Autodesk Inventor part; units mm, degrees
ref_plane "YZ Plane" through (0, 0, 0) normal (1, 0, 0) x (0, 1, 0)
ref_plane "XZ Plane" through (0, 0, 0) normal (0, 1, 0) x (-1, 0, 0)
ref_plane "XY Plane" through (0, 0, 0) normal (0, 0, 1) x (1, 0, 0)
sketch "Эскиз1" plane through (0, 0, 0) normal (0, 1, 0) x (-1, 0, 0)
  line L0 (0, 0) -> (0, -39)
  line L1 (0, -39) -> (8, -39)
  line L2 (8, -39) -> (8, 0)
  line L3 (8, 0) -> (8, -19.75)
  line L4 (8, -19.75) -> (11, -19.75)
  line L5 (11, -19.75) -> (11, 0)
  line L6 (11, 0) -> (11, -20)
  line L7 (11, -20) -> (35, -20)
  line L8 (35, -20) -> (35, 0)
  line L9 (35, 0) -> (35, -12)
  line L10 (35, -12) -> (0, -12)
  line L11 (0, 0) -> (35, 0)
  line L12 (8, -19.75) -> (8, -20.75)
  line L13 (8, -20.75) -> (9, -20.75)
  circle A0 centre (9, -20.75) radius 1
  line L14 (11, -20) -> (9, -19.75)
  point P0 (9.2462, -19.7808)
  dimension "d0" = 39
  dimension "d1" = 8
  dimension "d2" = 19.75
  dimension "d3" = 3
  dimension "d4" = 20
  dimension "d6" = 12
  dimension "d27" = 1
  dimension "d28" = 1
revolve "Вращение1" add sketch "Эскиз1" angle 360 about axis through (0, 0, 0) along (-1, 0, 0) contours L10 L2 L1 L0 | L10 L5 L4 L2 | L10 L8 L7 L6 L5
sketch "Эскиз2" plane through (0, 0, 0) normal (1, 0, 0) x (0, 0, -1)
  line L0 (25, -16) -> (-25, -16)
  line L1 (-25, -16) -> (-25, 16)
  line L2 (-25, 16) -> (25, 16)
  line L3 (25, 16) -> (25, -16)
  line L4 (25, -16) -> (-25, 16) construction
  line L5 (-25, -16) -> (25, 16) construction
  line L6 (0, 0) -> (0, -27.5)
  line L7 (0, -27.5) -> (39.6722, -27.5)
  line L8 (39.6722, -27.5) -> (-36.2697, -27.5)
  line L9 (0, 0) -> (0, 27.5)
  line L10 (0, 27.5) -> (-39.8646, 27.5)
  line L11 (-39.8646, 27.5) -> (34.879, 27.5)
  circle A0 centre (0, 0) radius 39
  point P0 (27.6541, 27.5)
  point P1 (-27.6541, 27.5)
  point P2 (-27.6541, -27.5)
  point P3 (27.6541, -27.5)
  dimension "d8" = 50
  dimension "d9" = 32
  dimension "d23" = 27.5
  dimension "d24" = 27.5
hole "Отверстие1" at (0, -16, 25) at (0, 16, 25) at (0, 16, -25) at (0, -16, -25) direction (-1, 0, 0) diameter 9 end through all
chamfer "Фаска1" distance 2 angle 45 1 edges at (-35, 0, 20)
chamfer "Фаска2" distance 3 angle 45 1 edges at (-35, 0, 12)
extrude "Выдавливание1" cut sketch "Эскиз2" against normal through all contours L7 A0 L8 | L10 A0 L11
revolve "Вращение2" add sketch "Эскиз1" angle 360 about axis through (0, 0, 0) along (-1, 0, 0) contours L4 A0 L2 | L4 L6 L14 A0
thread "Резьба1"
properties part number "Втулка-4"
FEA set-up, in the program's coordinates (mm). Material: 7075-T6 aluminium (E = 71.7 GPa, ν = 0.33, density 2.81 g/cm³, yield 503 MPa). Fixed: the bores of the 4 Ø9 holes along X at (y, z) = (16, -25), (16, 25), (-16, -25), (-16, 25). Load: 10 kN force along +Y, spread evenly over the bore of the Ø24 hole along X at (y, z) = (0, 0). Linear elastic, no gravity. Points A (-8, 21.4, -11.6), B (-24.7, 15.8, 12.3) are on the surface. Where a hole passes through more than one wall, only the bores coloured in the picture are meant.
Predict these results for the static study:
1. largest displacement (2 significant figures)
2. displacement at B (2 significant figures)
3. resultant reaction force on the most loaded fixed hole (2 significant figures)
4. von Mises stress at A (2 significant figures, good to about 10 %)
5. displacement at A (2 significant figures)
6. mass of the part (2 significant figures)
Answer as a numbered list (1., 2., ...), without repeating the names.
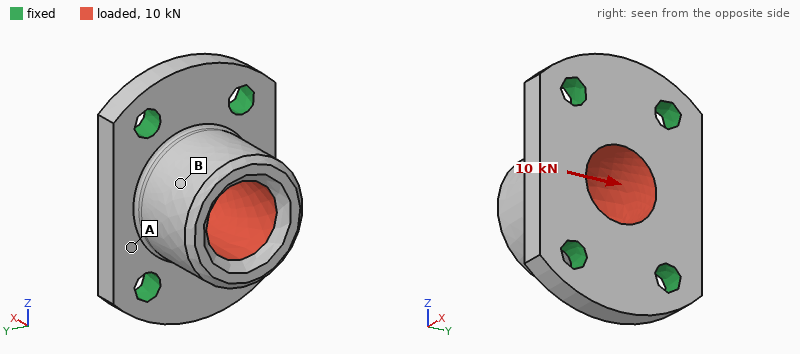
1. 35 µm
2. 26 µm
3. 3.3 kN
4. 20 MPa
5. 11 µm
6. 130 g
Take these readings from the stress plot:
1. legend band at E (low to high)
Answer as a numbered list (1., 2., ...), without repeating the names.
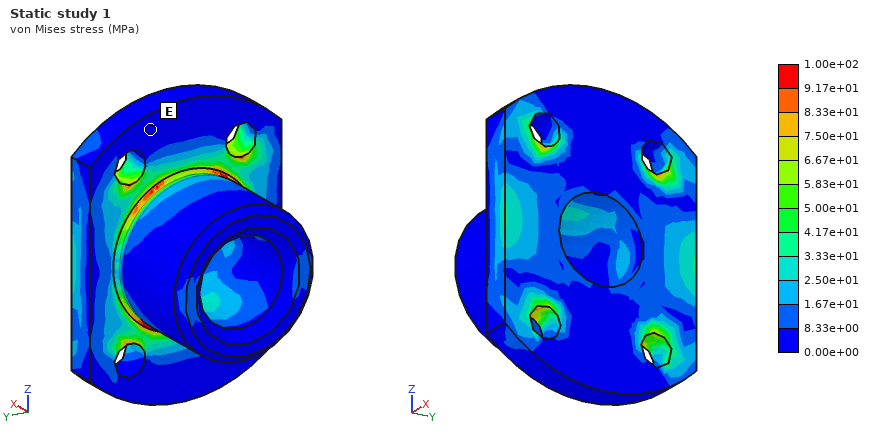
1. 0.00e+00 to 8.33e+00 MPa
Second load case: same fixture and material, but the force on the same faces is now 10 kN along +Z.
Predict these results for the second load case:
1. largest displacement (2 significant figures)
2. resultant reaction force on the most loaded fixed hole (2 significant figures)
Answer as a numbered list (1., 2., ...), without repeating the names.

1. 21 µm
2. 3.0 kN
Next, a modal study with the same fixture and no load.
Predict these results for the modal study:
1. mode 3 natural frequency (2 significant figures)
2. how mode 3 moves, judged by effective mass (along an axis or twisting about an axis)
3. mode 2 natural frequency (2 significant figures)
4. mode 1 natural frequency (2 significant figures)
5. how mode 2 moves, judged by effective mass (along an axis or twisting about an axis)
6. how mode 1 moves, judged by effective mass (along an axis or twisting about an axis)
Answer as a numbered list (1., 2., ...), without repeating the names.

1. 15 kHz
2. along X
3. 14 kHz
4. 10000 Hz
5. along Z
6. along Y
